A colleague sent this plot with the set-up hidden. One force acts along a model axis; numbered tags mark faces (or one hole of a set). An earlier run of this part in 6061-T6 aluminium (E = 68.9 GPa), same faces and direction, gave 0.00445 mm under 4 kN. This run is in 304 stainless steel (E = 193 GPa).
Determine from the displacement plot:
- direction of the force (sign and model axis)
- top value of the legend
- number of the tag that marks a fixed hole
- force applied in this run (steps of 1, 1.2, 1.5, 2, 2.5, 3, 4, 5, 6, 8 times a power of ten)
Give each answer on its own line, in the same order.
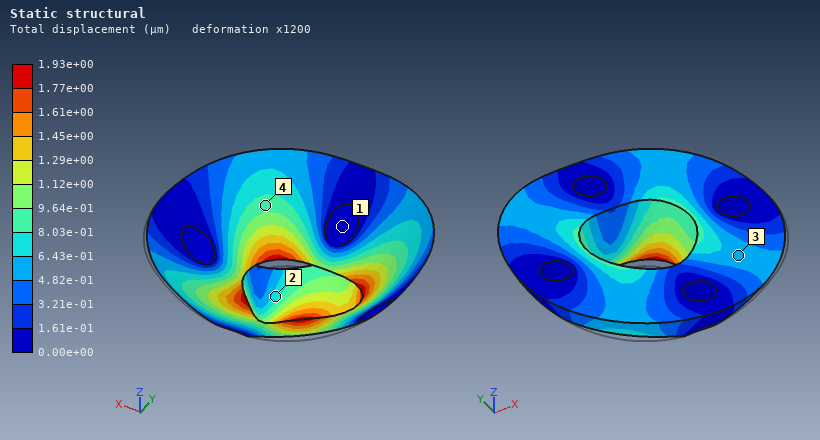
+Y
1.93e+00 µm
1
5 kN
